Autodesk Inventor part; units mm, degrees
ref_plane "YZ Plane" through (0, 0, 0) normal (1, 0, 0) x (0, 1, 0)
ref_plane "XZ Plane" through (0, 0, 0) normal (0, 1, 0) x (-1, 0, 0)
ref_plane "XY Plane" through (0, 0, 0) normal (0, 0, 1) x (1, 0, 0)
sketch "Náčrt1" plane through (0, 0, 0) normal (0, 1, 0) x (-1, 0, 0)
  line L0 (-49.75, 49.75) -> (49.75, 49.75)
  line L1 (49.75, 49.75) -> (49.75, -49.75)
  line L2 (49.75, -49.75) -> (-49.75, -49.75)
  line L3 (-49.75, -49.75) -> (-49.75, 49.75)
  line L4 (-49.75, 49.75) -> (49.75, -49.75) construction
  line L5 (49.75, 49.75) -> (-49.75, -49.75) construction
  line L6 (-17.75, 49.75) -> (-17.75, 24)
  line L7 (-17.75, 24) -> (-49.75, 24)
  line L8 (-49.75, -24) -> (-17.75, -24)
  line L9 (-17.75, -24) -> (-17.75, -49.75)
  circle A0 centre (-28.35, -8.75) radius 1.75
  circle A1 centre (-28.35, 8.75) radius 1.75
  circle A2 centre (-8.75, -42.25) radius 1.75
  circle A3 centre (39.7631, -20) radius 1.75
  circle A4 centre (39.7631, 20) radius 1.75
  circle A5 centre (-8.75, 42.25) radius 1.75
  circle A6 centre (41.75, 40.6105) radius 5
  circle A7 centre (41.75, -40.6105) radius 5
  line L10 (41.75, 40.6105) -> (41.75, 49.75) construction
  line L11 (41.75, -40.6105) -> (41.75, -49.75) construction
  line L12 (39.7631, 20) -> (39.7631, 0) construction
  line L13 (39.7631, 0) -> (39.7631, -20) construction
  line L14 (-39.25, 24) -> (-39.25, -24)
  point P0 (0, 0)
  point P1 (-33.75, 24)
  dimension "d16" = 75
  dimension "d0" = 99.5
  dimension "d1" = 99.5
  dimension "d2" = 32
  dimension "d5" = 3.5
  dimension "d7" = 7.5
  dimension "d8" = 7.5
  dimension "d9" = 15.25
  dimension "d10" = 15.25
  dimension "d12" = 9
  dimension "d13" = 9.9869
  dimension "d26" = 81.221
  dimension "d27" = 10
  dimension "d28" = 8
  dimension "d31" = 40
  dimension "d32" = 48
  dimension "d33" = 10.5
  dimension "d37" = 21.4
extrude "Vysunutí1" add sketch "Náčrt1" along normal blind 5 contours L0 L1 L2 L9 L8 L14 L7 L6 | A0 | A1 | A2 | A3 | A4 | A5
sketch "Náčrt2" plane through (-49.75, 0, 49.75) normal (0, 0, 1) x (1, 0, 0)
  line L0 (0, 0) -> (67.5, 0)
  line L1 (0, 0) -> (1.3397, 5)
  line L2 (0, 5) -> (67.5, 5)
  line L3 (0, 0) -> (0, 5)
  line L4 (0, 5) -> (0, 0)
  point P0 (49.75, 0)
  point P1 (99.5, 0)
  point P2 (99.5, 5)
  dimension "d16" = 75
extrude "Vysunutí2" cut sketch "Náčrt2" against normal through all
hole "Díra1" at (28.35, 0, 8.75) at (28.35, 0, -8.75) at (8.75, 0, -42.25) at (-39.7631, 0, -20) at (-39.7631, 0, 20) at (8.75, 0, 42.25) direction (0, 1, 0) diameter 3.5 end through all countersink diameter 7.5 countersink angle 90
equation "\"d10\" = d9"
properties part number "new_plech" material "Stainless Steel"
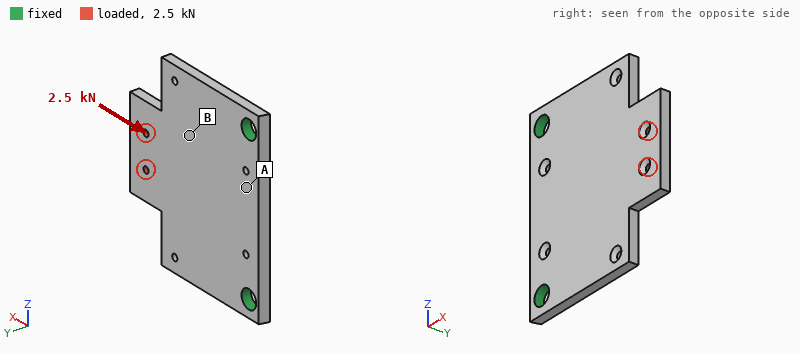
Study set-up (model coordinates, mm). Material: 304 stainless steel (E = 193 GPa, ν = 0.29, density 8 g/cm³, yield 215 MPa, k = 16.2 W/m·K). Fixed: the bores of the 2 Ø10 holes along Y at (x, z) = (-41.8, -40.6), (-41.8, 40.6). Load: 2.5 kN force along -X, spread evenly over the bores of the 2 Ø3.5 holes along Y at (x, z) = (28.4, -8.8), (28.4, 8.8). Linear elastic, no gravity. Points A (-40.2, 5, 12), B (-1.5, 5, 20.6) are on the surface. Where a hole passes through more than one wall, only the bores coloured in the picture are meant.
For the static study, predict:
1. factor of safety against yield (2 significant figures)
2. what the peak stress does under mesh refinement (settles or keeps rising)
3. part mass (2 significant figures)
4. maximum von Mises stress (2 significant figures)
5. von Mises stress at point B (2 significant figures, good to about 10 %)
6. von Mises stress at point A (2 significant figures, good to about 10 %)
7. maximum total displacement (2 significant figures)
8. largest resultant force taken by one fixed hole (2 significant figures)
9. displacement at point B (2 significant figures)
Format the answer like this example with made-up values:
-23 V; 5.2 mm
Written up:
3.0; settles; 300 g; 73 MPa; 14 MPa; 5.2 MPa; 53 µm; 1.3 kN; 13 µm
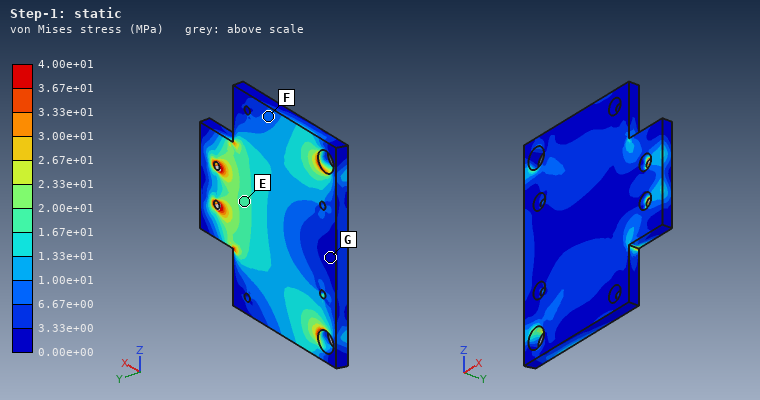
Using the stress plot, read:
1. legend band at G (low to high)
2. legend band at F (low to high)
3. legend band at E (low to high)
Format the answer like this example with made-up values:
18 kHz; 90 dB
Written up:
0.00e+00 to 3.33e+00 MPa; 6.67e+00 to 1.00e+01 MPa; 1.67e+01 to 2.00e+01 MPa
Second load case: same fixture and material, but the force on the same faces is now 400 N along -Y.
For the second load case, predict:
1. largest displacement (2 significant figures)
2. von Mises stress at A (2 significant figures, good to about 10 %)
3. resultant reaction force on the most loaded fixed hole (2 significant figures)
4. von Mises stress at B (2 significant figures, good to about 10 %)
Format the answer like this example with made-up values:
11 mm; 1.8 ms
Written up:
0.37 mm; 29 MPa; 200 N; 34 MPa
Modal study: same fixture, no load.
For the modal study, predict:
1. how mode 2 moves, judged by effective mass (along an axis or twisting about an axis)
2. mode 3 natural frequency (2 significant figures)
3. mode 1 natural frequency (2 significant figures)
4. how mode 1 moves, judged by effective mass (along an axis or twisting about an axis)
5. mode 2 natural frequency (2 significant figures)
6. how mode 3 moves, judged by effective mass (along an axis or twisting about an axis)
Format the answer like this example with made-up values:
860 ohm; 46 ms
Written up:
twisting about X; 3300 Hz; 680 Hz; along Y; 1900 Hz; along Y
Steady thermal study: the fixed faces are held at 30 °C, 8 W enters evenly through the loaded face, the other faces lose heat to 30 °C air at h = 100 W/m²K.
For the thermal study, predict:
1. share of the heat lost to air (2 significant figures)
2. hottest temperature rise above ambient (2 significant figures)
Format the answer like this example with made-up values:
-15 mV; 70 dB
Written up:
98 %; 37 K
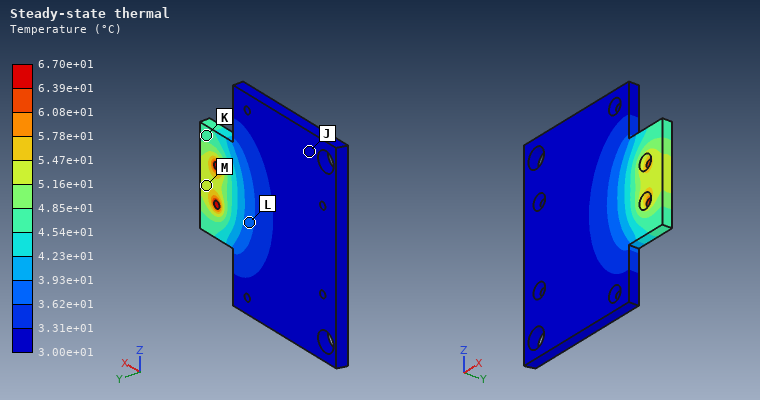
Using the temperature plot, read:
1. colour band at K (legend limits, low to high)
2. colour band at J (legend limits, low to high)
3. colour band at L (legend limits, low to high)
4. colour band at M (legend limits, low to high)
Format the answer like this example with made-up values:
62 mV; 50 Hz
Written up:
4.54e+01 to 4.85e+01 °C; 3.00e+01 to 3.31e+01 °C; 3.62e+01 to 3.93e+01 °C; 5.16e+01 to 5.47e+01 °C
